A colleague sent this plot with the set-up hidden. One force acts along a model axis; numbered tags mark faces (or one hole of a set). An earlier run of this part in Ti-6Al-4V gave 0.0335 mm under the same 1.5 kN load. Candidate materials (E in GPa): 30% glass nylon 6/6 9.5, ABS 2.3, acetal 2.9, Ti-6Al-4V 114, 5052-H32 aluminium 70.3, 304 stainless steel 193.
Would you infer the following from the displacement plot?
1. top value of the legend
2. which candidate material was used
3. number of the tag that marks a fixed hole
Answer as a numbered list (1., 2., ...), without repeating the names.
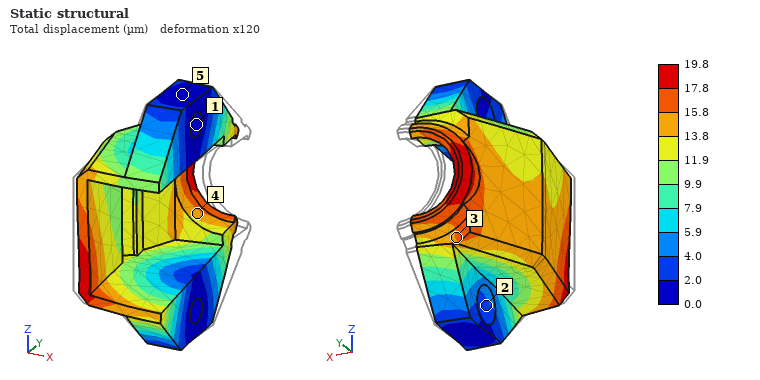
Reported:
1. 19.8 µm
2. 304 stainless steel
3. 1
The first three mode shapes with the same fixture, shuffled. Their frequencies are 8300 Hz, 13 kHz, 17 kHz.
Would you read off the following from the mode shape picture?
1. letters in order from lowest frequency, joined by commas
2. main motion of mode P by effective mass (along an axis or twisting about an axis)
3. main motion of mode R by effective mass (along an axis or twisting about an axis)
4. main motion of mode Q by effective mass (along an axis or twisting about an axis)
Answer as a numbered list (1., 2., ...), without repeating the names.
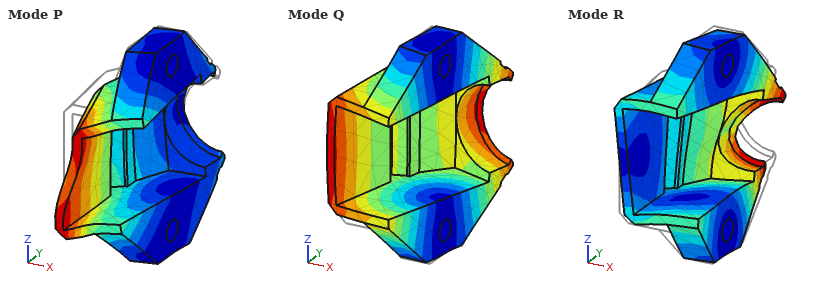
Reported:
1. Q, P, R
2. along Z
3. along Z
4. along Y
